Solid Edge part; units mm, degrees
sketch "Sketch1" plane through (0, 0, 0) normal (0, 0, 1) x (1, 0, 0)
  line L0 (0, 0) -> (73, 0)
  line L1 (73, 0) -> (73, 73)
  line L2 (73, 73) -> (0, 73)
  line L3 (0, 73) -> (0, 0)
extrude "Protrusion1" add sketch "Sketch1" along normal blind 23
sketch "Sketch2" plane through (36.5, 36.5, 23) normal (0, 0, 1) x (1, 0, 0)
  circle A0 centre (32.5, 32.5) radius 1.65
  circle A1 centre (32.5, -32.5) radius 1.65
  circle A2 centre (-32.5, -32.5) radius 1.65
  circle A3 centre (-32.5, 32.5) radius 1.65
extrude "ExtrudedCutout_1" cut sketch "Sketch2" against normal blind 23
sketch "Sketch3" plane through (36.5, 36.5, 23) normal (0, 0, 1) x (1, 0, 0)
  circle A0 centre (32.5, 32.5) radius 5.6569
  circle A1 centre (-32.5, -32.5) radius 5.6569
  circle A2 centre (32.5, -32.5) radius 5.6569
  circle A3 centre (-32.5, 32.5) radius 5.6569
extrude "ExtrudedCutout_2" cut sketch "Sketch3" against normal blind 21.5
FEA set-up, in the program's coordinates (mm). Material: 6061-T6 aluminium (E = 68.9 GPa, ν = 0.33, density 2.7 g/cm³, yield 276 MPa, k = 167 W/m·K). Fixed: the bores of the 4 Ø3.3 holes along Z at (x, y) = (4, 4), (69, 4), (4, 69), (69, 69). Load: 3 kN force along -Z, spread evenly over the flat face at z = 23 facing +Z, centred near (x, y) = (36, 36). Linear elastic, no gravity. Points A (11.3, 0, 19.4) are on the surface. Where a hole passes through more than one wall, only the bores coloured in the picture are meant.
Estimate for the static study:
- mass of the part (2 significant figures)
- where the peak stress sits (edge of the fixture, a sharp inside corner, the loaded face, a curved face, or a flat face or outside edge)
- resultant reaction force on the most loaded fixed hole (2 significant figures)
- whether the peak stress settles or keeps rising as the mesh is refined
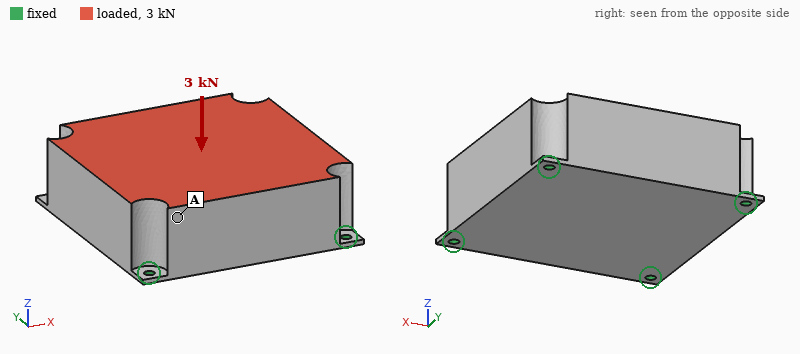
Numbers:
310 g
edge of the fixture
840 N
keeps rising
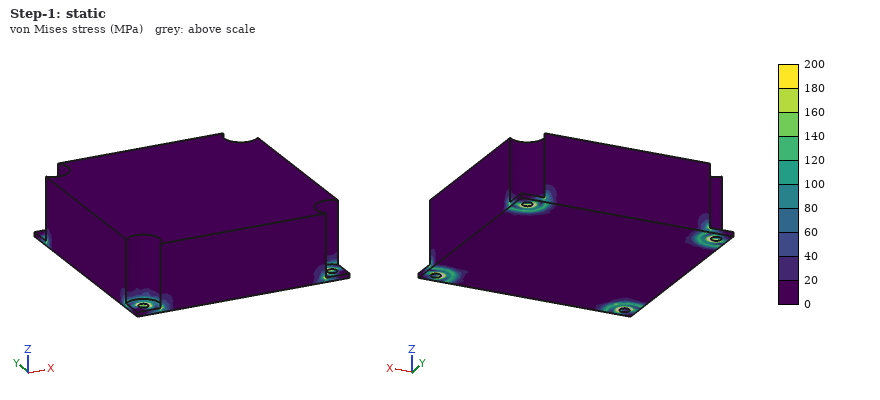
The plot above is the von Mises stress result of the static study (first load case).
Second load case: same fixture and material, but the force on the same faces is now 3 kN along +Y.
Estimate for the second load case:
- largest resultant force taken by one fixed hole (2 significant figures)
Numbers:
960 N
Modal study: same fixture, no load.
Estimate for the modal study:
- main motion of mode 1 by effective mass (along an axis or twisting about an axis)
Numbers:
along Z
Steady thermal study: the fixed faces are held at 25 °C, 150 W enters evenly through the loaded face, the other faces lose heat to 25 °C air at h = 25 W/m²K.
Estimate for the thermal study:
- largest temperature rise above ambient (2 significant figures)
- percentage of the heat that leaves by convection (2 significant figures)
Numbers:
66 K
12 %
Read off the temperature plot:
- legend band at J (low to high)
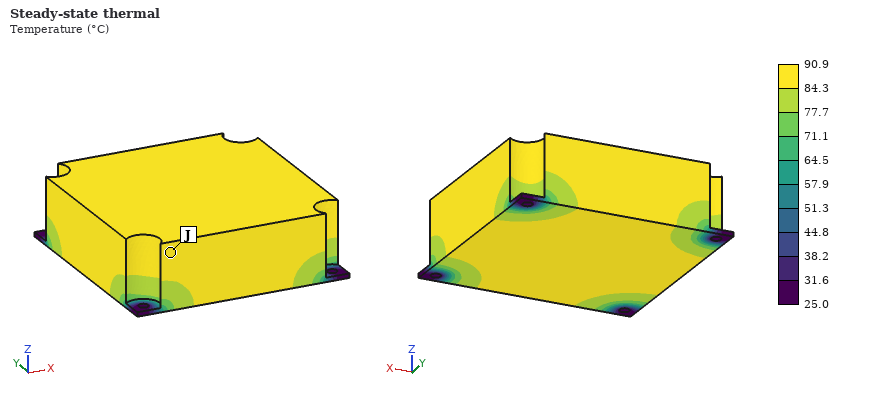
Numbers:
84.3 to 90.9 °C
